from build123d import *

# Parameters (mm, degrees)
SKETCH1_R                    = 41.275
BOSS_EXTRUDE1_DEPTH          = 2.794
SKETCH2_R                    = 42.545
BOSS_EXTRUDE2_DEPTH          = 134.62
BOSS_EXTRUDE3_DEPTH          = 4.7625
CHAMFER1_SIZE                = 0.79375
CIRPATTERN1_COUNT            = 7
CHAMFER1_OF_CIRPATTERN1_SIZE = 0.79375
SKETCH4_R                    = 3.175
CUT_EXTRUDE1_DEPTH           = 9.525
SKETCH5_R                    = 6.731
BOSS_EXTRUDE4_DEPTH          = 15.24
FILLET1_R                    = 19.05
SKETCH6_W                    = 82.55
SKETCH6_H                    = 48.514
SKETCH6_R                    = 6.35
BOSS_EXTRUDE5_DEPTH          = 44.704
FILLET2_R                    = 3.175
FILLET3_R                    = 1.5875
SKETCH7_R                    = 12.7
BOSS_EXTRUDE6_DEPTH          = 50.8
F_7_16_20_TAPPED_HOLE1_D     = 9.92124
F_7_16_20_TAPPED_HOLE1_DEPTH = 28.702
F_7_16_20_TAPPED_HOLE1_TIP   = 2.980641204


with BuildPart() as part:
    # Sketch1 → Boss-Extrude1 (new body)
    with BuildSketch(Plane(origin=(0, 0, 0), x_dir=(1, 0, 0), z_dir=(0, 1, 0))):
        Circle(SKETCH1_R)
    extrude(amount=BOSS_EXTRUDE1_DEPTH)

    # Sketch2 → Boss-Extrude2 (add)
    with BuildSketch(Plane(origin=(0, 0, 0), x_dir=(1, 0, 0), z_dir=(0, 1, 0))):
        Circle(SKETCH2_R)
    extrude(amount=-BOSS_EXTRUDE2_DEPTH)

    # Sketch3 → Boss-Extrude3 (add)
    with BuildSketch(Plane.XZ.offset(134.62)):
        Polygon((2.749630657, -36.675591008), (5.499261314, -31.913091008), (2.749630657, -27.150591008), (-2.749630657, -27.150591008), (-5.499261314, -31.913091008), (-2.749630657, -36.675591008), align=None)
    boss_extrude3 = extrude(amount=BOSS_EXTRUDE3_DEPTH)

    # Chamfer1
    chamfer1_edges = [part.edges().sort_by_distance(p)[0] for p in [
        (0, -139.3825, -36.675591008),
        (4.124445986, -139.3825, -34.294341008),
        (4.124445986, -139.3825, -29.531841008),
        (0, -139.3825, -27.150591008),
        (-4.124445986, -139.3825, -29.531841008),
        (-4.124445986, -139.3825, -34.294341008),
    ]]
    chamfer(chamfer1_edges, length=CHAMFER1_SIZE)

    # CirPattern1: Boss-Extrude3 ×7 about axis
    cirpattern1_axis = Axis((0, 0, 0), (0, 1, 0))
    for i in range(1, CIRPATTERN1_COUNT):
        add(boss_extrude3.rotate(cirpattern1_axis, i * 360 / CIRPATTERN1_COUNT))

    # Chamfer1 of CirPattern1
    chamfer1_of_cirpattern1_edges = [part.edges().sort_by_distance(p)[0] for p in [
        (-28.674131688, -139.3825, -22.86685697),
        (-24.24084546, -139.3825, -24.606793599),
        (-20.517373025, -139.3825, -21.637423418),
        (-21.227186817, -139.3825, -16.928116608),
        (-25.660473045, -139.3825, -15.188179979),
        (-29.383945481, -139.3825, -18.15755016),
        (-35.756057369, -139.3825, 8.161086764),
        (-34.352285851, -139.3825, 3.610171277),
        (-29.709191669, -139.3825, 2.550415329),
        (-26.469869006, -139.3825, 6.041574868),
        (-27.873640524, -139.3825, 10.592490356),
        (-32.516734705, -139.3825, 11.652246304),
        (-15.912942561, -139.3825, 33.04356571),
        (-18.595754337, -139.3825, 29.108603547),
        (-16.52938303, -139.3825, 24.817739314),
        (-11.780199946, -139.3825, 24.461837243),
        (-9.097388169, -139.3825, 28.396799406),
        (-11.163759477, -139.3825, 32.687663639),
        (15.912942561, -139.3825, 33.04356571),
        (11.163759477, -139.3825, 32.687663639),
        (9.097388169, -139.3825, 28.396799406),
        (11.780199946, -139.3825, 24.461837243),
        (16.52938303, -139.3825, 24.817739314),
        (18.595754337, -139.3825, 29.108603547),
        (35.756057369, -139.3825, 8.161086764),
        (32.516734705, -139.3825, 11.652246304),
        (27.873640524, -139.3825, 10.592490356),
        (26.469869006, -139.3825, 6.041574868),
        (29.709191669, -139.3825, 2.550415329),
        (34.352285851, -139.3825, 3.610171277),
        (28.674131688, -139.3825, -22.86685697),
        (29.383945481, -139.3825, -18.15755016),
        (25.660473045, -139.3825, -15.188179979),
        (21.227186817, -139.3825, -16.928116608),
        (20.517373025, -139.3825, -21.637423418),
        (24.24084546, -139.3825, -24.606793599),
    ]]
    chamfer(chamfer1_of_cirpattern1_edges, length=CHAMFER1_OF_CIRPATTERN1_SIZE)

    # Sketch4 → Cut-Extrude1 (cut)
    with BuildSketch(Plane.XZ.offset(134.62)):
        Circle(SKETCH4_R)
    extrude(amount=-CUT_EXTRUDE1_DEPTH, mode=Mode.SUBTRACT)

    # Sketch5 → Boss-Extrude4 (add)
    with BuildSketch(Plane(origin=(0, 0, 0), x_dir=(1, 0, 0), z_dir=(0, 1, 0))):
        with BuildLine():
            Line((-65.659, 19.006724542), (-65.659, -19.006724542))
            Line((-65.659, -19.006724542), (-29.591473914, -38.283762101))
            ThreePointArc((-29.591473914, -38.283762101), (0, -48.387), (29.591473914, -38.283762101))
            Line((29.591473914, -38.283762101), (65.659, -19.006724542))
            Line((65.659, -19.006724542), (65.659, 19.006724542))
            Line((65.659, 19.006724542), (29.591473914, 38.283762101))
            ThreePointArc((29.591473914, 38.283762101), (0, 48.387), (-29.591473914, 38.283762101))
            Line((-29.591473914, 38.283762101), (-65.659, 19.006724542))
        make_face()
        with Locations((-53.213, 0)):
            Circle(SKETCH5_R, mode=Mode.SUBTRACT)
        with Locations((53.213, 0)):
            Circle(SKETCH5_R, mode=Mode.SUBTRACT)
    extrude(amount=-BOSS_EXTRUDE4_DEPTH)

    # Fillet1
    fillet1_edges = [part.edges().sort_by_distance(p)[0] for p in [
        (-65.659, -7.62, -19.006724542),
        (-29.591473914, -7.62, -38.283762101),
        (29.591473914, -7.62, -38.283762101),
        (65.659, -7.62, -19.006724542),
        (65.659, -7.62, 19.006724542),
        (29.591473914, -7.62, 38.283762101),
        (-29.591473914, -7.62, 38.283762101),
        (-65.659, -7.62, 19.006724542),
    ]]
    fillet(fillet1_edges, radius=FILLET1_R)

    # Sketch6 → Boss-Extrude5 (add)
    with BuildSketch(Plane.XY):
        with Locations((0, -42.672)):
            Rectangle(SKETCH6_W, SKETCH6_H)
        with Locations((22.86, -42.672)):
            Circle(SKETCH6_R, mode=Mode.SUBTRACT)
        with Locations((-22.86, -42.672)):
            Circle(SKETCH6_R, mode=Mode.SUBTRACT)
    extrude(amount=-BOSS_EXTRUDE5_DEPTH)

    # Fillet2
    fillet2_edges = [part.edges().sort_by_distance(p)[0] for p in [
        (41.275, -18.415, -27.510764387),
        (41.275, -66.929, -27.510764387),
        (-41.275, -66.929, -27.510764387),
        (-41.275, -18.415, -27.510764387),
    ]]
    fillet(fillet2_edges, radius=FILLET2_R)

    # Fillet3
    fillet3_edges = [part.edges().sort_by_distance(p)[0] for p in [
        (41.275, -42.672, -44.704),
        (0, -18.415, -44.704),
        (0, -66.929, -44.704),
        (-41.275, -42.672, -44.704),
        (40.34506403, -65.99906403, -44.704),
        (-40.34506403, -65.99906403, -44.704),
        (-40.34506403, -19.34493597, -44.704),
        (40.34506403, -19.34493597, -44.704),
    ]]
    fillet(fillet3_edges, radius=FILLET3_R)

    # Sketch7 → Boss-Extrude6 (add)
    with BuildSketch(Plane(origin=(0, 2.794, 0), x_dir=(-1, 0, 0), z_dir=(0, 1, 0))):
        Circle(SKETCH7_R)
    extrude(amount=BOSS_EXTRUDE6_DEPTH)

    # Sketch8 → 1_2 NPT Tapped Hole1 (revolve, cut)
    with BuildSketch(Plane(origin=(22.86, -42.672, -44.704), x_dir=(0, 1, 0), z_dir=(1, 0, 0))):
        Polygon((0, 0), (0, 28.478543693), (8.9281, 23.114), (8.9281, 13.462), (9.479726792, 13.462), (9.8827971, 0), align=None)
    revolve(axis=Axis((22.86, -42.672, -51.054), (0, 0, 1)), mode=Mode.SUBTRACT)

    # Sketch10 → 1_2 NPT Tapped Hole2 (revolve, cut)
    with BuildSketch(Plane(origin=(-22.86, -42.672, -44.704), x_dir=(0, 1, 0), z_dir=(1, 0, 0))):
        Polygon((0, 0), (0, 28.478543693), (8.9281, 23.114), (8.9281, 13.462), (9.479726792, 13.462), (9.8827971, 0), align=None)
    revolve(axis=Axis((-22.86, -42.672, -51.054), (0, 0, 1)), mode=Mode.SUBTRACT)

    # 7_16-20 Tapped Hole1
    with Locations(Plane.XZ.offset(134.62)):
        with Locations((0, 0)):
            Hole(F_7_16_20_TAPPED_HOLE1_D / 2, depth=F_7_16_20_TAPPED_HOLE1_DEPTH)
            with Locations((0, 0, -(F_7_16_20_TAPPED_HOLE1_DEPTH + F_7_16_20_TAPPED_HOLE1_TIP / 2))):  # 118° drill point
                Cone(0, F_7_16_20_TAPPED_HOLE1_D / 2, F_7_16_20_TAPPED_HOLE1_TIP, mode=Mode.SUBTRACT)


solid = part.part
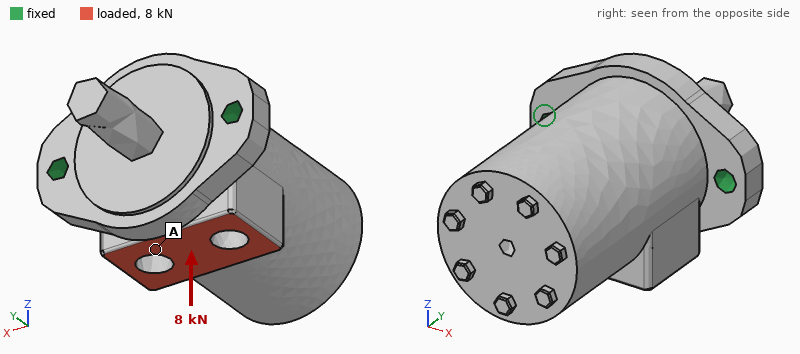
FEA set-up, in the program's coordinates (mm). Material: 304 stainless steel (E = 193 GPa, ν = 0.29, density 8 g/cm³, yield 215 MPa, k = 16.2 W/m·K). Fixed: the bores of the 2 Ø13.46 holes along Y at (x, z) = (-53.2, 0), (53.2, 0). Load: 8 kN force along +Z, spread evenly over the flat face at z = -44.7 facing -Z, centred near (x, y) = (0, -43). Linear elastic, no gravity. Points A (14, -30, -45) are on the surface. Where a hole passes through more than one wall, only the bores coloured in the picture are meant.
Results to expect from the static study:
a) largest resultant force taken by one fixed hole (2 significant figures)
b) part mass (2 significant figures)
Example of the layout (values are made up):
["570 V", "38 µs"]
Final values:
["4.0 kN", "7.1 kg"]
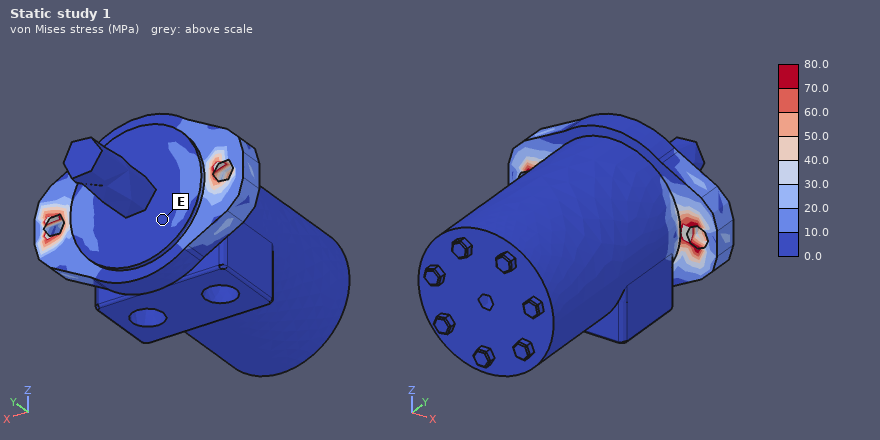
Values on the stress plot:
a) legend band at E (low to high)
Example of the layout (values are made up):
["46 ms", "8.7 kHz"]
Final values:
["0.0 to 10.0 MPa"]
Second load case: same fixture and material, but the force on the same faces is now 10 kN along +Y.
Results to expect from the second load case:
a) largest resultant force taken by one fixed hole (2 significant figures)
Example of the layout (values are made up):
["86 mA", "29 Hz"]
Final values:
["5.3 kN"]
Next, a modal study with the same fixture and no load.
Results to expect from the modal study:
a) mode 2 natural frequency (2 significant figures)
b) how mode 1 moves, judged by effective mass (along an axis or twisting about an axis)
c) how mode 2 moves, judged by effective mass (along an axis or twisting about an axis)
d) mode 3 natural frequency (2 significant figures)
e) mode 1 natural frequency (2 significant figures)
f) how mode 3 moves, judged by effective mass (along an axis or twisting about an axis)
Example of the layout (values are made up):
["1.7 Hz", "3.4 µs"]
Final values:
["2000 Hz", "along Z", "along X", "3400 Hz", "630 Hz", "along Y"]
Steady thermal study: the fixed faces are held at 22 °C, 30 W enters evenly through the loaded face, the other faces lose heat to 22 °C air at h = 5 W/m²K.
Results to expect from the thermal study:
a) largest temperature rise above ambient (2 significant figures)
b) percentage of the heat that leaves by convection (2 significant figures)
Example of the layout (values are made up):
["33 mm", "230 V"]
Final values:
["39 K", "24 %"]
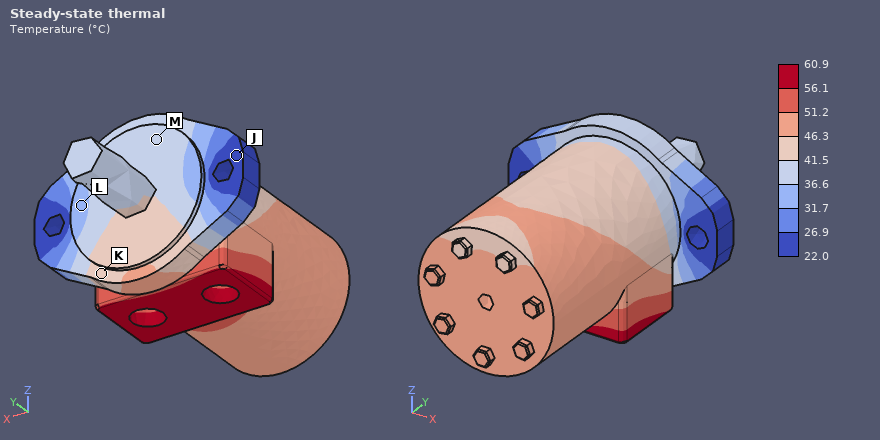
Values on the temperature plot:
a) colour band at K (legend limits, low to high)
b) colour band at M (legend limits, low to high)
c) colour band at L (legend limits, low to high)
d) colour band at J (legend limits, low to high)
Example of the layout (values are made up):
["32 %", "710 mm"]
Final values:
["41.5 to 46.3 °C", "36.6 to 41.5 °C", "31.7 to 36.6 °C", "22.0 to 26.9 °C"]
